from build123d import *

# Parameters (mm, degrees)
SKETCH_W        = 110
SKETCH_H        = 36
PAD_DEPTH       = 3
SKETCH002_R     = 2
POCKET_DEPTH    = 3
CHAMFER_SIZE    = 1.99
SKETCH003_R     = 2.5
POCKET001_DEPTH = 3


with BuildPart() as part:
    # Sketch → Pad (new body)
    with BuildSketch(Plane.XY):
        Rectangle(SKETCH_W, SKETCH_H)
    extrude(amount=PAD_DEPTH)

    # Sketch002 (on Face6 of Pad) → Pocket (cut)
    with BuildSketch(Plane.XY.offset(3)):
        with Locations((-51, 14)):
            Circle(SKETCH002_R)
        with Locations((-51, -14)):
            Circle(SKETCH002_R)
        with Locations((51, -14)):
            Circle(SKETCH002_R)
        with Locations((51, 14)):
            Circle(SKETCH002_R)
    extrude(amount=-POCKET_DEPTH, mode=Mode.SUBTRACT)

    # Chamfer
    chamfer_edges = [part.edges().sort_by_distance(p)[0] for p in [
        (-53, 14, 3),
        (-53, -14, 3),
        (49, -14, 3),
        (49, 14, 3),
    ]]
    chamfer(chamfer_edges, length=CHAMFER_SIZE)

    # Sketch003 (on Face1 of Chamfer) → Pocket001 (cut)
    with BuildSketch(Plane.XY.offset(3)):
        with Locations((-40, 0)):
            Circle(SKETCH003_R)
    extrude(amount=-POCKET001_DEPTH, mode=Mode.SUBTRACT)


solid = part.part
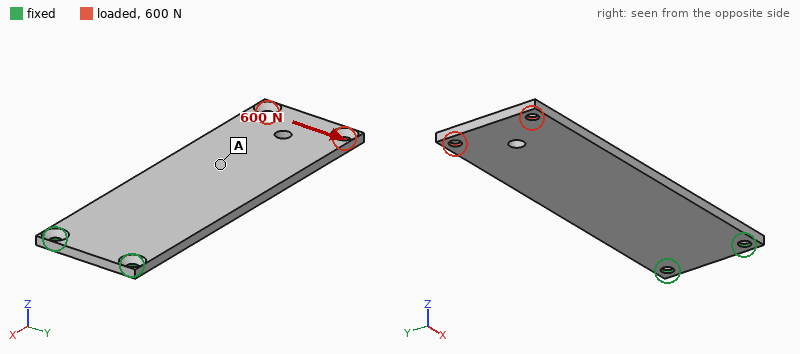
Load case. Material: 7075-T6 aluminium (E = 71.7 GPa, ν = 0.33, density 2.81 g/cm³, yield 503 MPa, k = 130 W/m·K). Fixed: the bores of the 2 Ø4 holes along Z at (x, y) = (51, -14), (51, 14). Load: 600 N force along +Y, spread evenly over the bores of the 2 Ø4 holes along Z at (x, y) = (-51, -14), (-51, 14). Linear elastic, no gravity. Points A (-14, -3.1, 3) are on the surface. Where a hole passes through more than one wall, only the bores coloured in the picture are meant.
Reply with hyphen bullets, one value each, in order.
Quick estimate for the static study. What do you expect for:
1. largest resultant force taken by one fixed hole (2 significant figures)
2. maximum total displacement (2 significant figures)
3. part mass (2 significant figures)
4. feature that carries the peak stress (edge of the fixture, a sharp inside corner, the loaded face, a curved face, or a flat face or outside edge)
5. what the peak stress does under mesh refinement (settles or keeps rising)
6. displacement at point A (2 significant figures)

- 2.1 kN
- 0.41 mm
- 32 g
- edge of the fixture
- keeps rising
- 0.16 mm
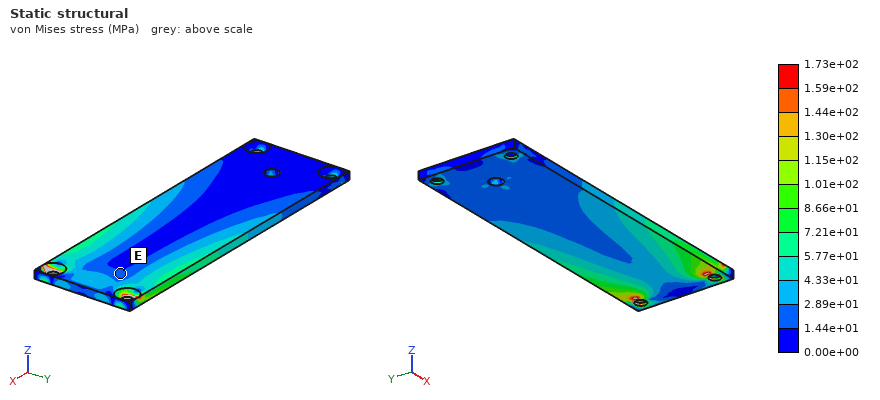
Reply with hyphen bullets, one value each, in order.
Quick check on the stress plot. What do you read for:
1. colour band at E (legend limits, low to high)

- 1.44e+01 to 2.89e+01 MPa
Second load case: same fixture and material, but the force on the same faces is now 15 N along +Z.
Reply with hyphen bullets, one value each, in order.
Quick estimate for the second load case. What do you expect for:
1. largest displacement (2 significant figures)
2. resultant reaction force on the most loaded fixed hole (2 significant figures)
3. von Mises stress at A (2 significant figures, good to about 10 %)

- 1.2 mm
- 9.2 N
- 10 MPa
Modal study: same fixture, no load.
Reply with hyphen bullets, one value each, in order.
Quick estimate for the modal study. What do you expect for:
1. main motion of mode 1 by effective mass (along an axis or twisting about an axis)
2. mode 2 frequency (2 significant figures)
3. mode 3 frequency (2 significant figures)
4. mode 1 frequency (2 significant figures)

- along Z
- 1300 Hz
- 1300 Hz
- 190 Hz
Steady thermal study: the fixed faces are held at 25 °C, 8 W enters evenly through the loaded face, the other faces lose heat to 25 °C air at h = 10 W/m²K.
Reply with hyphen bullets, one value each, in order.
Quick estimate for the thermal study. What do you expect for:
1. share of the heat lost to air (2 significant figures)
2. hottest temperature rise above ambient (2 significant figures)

- 27 %
- 57 K
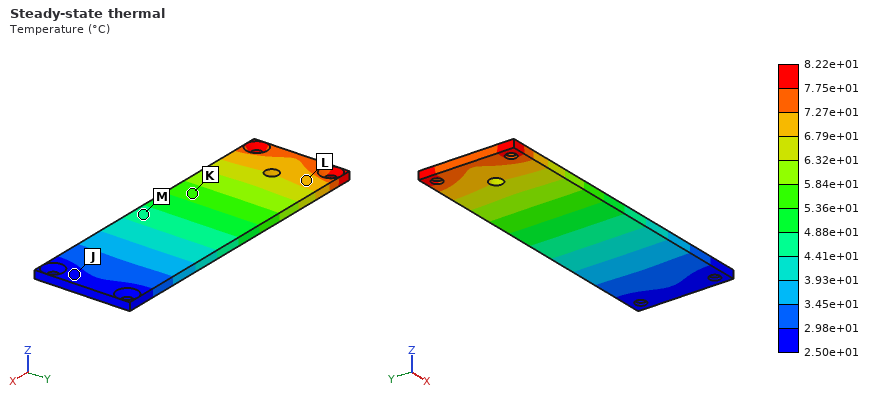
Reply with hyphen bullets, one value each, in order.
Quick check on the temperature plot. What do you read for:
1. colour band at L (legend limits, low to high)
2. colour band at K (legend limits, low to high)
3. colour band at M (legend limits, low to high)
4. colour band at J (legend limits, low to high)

- 6.79e+01 to 7.27e+01 °C
- 5.36e+01 to 5.84e+01 °C
- 4.41e+01 to 4.88e+01 °C
- 2.50e+01 to 2.98e+01 °C
